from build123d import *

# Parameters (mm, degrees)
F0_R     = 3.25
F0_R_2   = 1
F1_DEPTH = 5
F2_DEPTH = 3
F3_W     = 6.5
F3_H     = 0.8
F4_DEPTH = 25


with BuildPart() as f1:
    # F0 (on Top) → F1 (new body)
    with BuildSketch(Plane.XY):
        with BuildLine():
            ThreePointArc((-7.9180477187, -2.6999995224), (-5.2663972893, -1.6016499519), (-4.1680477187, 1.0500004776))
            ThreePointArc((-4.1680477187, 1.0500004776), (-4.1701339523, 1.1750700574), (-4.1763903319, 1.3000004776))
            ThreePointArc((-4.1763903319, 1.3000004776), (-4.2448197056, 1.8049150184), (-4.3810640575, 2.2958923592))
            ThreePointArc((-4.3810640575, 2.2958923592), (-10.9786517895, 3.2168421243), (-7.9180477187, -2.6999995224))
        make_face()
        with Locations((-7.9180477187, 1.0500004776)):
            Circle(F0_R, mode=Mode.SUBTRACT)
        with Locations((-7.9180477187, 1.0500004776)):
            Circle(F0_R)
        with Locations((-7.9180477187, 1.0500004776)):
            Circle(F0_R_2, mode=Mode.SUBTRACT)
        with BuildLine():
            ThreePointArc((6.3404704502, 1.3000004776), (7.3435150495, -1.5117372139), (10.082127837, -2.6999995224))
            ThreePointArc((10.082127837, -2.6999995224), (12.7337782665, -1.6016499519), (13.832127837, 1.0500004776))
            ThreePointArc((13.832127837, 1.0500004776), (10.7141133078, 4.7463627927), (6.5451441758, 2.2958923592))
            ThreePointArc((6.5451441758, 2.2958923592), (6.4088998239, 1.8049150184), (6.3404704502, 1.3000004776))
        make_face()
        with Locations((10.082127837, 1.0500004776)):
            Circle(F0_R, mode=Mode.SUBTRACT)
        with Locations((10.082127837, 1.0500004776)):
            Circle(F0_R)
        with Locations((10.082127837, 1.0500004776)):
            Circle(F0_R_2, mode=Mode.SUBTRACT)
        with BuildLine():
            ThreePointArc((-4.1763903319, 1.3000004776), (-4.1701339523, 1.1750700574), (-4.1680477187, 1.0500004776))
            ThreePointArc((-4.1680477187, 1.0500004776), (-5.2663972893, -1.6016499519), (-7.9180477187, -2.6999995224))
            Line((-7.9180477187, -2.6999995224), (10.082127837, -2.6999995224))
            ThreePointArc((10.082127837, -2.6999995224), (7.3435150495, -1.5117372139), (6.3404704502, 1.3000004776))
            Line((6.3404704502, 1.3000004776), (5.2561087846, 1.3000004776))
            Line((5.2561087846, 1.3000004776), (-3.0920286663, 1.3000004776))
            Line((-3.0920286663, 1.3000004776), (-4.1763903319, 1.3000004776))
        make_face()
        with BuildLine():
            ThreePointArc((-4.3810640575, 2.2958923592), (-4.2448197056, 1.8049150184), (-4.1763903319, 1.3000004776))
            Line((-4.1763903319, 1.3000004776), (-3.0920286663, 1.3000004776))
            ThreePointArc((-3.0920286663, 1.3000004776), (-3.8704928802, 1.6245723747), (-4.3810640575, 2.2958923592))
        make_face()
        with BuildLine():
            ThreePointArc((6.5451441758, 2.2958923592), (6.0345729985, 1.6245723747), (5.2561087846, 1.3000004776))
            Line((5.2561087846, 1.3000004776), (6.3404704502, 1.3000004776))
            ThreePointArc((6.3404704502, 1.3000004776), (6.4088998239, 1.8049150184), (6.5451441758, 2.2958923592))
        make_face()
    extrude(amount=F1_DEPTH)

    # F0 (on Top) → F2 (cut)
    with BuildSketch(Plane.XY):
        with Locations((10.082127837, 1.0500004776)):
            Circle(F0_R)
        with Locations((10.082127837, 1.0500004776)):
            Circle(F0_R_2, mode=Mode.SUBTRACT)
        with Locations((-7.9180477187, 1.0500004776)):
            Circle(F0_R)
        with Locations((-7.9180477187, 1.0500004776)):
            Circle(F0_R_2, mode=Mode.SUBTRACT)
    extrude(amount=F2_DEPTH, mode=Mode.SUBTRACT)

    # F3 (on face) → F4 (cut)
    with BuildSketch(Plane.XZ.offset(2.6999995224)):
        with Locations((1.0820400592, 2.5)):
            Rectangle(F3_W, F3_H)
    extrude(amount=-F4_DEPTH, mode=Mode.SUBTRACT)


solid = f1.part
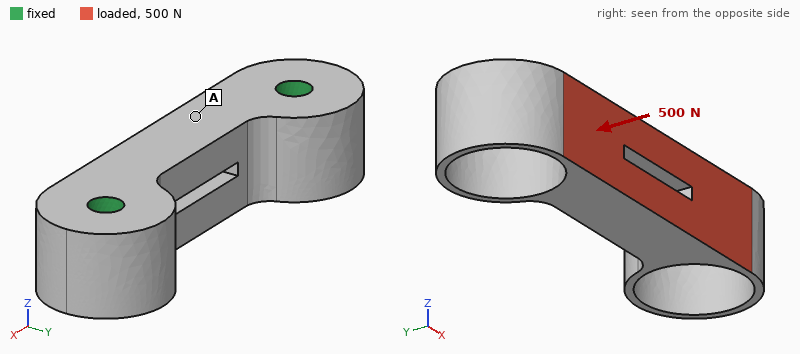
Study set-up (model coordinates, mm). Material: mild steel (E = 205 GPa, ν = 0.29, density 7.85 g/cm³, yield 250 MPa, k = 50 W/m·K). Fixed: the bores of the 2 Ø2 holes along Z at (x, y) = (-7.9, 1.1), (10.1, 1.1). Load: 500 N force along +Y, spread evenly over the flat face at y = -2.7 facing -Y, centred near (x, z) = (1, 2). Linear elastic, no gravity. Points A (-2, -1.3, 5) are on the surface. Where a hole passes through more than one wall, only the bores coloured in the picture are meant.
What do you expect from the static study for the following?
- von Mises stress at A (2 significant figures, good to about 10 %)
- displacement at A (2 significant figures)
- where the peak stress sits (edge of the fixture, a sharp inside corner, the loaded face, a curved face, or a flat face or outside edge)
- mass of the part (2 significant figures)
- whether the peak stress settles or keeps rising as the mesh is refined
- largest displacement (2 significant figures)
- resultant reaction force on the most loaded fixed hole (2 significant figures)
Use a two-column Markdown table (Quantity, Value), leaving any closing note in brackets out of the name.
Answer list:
| Quantity | Value |
|---|---|
| von Mises stress at A | 24 MPa |
| displacement at A | 2.2 µm |
| where the peak stress sits | edge of the fixture |
| mass of the part | 3.6 g |
| whether the peak stress settles or keeps rising as the mesh is refined | keeps rising |
| largest displacement | 5.5 µm |
| resultant reaction force on the most loaded fixed hole | 280 N |
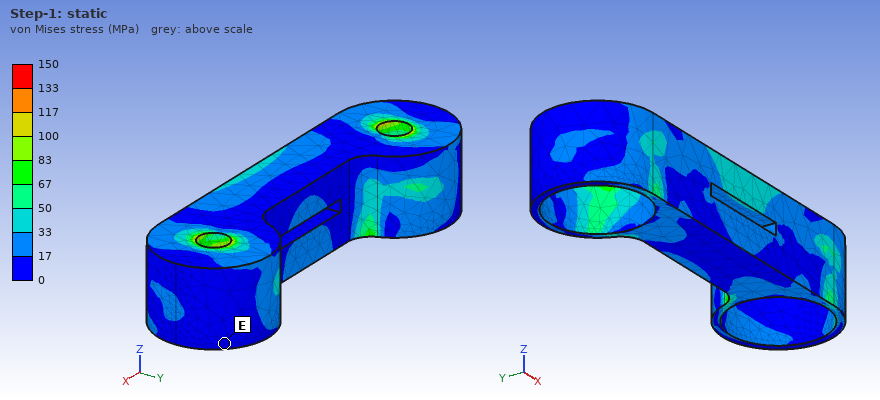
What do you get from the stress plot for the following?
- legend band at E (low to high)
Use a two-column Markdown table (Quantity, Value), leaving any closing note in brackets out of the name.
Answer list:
| Quantity | Value |
|---|---|
| legend band at E | 0 to 17 MPa |
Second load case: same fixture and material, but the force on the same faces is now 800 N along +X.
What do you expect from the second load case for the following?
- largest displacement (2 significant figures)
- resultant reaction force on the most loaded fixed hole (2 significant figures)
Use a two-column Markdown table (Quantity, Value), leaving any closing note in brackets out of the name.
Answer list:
| Quantity | Value |
|---|---|
| largest displacement | 2.3 µm |
| resultant reaction force on the most loaded fixed hole | 430 N |
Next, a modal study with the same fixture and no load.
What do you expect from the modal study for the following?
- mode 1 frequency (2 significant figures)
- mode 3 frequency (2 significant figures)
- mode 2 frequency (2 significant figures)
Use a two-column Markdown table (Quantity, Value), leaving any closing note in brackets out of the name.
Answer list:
| Quantity | Value |
|---|---|
| mode 1 frequency | 34 kHz |
| mode 3 frequency | 62 kHz |
| mode 2 frequency | 48 kHz |
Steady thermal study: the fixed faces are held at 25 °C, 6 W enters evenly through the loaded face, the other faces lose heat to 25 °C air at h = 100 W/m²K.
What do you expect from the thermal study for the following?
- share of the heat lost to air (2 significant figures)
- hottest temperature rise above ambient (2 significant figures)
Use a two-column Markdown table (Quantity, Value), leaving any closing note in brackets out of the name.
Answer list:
| Quantity | Value |
|---|---|
| share of the heat lost to air | 9.7 % |
| hottest temperature rise above ambient | 21 K |
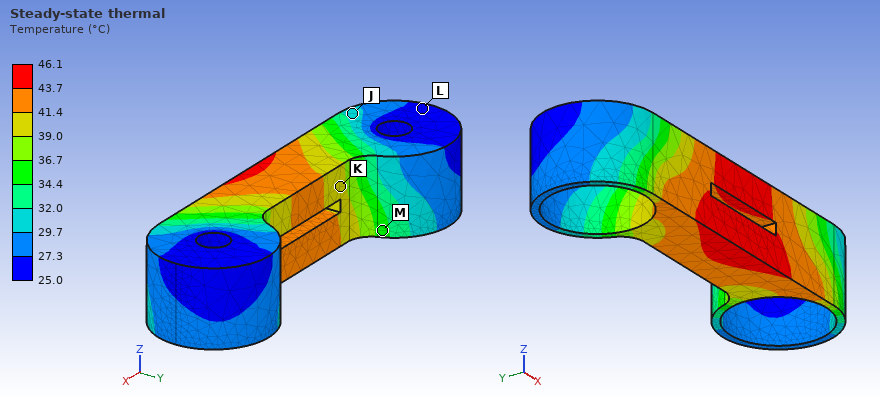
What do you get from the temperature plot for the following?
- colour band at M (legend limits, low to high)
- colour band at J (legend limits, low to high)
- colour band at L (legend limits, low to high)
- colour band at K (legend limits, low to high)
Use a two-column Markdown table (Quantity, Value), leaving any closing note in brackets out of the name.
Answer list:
| Quantity | Value |
|---|---|
| colour band at M | 34.4 to 36.7 °C |
| colour band at J | 29.7 to 32.0 °C |
| colour band at L | 25.0 to 27.3 °C |
| colour band at K | 39.0 to 41.4 °C |
